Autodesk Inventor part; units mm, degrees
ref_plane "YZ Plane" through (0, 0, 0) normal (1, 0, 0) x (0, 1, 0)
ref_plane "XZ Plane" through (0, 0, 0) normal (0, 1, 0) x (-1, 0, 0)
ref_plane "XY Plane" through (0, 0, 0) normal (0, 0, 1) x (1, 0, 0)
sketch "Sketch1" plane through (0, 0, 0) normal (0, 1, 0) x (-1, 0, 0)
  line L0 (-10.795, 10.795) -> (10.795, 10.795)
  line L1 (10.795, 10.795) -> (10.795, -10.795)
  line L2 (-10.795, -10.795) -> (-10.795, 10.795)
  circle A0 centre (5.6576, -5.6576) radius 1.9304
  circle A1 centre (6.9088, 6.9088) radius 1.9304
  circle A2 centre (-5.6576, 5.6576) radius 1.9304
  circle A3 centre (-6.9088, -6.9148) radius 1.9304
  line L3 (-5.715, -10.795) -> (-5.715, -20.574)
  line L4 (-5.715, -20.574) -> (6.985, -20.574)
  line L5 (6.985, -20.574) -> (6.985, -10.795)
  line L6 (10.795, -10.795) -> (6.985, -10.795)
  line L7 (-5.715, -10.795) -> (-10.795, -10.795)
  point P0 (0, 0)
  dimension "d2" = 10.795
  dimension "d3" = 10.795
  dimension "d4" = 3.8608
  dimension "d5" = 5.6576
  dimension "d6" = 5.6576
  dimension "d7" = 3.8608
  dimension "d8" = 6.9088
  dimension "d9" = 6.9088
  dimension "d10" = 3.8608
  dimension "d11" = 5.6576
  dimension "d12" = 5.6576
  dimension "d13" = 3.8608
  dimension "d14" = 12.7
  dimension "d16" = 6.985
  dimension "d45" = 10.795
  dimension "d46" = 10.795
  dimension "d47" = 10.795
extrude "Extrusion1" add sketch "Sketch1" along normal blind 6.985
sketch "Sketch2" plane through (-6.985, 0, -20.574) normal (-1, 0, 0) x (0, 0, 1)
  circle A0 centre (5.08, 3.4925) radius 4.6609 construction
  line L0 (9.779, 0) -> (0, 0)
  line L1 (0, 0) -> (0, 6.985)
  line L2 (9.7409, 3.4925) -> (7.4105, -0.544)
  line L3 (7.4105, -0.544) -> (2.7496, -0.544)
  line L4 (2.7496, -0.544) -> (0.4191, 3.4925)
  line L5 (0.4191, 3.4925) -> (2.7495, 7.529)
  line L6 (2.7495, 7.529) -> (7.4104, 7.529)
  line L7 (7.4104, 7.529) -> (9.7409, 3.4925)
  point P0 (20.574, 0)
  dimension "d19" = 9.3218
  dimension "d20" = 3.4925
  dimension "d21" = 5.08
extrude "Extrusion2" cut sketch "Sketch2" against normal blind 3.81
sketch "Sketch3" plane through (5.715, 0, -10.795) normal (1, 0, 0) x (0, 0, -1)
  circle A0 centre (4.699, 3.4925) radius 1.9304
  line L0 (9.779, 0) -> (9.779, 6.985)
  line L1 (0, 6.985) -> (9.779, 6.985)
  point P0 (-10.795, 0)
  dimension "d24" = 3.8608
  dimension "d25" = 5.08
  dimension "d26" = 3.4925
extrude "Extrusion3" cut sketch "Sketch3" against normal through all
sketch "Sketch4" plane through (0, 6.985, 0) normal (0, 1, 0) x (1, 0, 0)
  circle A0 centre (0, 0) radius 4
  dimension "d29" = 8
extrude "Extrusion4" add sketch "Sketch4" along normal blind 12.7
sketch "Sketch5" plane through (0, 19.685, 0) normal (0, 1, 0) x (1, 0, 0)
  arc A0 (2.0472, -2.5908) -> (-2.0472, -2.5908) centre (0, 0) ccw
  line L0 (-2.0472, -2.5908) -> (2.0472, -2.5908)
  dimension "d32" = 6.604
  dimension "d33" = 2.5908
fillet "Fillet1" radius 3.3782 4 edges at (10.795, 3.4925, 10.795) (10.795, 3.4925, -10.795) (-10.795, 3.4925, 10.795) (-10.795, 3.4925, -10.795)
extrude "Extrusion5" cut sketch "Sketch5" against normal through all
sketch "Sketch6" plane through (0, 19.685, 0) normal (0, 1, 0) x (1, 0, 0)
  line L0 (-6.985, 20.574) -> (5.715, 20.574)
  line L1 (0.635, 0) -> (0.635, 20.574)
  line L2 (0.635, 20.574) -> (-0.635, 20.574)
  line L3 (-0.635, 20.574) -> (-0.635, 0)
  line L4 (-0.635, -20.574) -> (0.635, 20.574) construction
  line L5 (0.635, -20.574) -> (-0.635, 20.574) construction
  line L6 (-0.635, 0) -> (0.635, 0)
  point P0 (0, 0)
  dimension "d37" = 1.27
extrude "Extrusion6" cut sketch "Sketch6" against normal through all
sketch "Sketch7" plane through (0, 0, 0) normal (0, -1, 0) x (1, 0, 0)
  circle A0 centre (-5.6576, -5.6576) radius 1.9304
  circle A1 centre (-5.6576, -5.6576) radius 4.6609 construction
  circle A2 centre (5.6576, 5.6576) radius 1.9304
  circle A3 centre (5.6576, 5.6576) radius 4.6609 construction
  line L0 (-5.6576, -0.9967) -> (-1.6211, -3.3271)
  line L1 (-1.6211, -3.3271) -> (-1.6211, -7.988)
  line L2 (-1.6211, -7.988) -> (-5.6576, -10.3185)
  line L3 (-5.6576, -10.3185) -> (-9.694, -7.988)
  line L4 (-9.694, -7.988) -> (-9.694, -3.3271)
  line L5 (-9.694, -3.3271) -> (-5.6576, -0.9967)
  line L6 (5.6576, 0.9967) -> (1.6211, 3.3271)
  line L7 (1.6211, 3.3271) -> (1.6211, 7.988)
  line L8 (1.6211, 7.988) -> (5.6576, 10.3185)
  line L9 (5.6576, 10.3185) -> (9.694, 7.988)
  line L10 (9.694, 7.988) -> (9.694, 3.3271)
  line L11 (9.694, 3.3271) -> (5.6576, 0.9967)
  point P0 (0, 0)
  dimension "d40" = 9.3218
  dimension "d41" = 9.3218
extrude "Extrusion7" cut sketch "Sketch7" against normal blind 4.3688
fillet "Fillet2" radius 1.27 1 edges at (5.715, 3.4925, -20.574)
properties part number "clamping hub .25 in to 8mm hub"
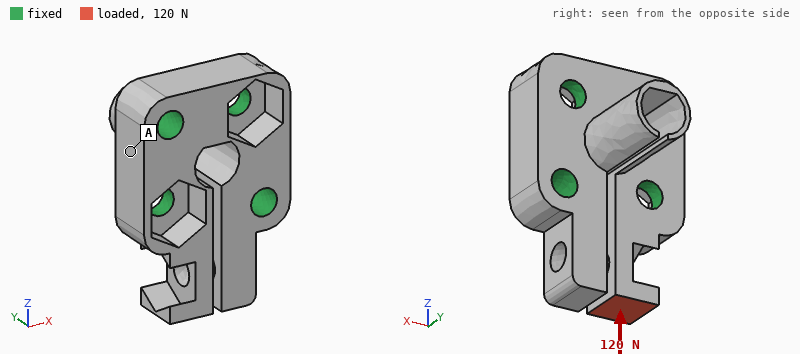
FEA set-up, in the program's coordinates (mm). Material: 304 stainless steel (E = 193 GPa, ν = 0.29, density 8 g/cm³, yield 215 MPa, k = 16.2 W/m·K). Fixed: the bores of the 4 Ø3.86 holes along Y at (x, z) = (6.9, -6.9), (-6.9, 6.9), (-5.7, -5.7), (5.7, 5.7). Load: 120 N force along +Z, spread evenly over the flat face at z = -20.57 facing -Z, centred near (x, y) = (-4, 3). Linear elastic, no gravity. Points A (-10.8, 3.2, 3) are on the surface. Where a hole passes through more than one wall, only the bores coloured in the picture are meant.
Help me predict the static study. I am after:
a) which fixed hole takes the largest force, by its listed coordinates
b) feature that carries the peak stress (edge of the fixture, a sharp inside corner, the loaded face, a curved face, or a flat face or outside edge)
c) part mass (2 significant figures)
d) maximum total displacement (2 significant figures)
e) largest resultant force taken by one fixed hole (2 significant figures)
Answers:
(-5.7, -5.7)
a curved face
23 g
15 µm
110 N
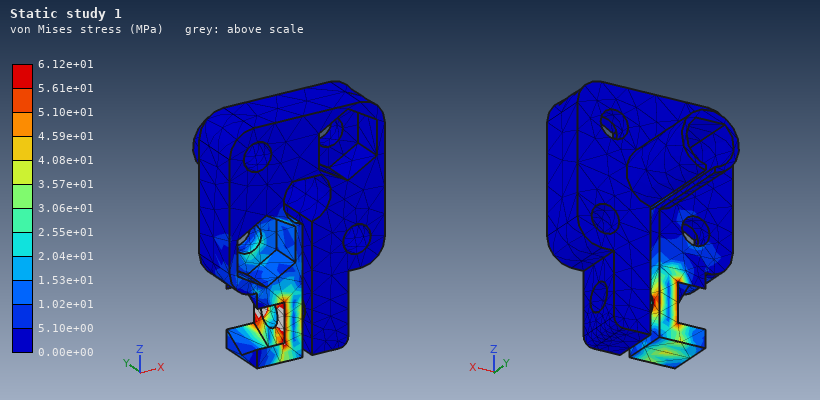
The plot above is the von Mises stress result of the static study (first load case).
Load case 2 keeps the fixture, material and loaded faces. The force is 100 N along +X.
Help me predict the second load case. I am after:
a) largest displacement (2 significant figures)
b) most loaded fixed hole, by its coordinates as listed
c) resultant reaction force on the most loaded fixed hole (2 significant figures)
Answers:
38 µm
(-5.7, -5.7)
150 N
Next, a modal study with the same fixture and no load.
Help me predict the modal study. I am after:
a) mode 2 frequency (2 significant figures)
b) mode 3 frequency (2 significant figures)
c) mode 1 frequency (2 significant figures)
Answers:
13 kHz
13 kHz
11 kHz
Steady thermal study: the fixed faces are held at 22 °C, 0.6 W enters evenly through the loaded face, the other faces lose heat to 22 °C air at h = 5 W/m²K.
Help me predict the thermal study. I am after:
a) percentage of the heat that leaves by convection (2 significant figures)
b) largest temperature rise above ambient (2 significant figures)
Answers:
6.1 %
40 K
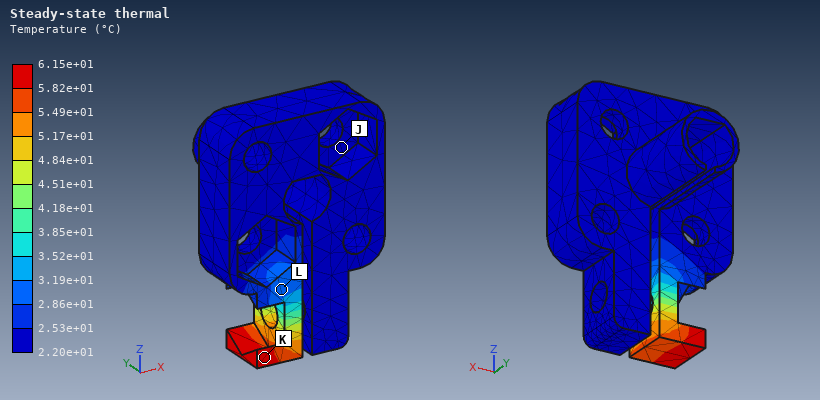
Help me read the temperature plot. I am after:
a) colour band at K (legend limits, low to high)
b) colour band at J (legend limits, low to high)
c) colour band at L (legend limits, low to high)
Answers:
5.82e+01 to 6.15e+01 °C
2.20e+01 to 2.53e+01 °C
2.86e+01 to 3.19e+01 °C
